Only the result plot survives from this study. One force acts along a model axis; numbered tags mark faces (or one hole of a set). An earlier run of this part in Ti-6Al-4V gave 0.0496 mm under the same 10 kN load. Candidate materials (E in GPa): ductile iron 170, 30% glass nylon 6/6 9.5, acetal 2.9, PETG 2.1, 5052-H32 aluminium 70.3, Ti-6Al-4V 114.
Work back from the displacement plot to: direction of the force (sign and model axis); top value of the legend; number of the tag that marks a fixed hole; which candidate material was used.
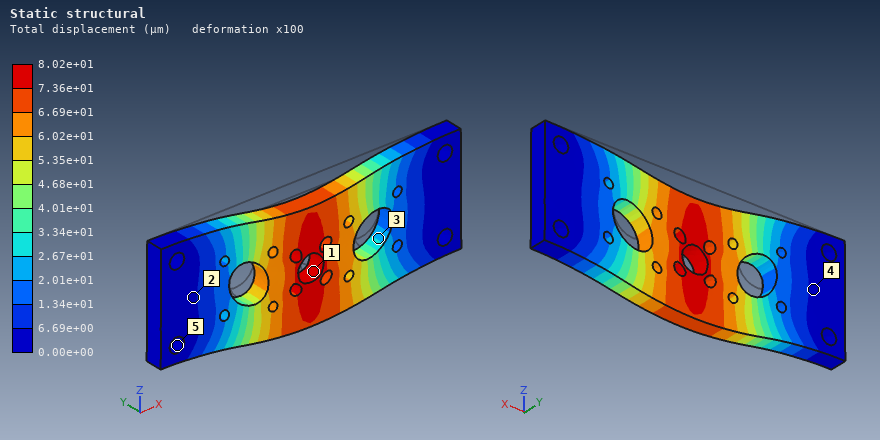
-Z
8.02e+01 µm
5
5052-H32 aluminium
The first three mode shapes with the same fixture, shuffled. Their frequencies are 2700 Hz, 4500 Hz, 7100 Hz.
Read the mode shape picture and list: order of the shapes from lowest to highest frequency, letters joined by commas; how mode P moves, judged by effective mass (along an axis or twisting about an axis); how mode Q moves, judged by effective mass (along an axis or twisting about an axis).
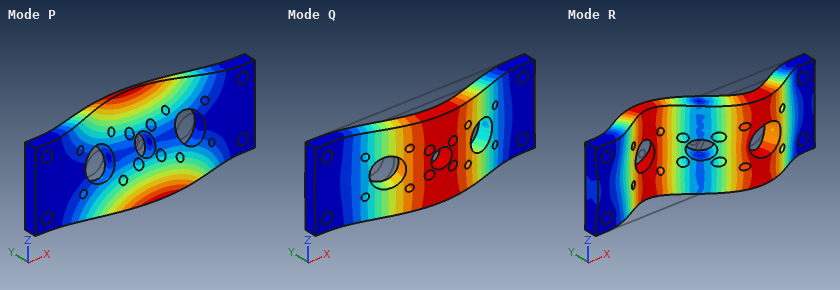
Q, P, R
twisting about X
along Y
